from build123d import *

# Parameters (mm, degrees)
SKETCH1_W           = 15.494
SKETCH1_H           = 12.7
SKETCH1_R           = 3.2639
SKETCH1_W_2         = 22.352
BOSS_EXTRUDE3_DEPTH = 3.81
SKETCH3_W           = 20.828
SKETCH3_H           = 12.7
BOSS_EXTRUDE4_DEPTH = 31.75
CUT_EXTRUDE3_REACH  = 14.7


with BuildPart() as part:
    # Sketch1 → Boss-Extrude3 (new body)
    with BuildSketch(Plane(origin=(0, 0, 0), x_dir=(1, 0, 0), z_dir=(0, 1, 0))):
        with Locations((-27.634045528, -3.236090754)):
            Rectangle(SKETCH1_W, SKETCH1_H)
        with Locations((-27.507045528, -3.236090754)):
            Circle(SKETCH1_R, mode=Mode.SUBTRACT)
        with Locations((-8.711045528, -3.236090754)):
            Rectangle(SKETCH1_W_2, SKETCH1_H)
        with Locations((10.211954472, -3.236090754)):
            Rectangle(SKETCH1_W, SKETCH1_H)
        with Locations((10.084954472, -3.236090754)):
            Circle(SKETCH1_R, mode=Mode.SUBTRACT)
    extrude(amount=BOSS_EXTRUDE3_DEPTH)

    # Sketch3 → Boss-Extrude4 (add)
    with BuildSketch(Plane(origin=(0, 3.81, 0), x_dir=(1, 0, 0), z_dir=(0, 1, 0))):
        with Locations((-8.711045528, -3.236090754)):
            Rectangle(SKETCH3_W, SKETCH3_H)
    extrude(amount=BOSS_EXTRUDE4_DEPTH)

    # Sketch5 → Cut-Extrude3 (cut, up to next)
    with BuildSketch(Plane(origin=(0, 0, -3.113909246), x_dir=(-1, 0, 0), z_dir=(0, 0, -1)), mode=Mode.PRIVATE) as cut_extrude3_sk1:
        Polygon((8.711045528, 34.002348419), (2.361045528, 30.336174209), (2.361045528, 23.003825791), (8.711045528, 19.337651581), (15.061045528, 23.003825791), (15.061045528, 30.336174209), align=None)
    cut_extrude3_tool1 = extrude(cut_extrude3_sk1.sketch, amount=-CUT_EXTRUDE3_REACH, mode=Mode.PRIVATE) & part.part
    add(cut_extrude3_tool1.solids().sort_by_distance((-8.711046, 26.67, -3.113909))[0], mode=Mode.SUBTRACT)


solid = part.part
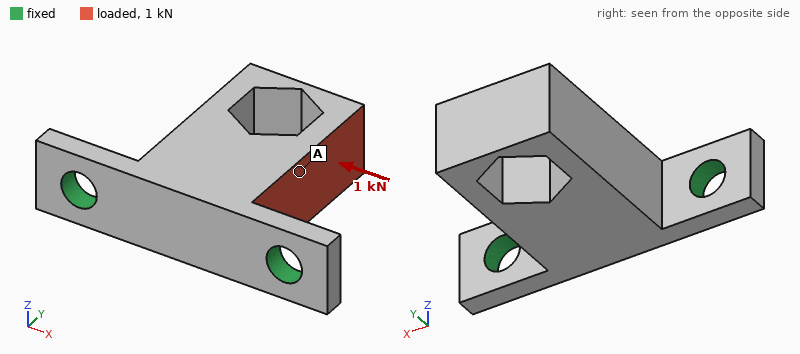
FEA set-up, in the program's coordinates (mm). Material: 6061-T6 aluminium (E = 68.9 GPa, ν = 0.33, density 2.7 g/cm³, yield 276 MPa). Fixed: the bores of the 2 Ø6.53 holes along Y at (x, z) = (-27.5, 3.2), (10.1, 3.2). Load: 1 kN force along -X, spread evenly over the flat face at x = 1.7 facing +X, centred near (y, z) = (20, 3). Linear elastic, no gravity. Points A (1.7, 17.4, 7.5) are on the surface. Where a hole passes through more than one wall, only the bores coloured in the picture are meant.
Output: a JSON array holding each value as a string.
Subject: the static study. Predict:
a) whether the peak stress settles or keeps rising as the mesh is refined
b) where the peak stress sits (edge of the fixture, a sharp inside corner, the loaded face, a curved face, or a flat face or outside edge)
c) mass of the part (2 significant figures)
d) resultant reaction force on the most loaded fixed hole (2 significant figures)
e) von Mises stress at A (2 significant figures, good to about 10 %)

["keeps rising", "edge of the fixture", "24 g", "840 N", "15 MPa"]
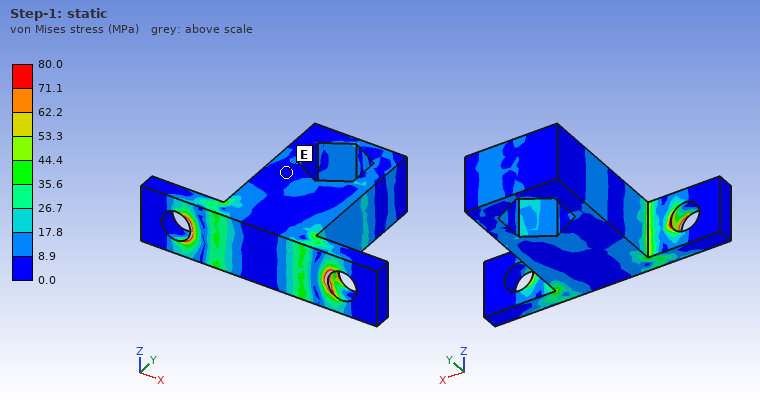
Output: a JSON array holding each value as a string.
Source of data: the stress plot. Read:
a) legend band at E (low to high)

["0.0 to 8.9 MPa"]
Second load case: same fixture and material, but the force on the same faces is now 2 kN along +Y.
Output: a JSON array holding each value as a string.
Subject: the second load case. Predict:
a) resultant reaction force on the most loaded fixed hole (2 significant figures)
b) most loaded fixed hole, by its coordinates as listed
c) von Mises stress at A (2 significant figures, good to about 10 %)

["1.8 kN", "(10.1, 3.2)", "28 MPa"]
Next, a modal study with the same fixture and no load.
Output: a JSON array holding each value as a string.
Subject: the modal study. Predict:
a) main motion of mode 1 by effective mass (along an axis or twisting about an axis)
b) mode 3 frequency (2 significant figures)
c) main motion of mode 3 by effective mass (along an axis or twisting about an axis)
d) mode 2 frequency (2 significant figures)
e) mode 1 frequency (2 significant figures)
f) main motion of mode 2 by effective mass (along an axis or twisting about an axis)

["along Z", "11 kHz", "along Y", "7200 Hz", "2700 Hz", "along X"]
